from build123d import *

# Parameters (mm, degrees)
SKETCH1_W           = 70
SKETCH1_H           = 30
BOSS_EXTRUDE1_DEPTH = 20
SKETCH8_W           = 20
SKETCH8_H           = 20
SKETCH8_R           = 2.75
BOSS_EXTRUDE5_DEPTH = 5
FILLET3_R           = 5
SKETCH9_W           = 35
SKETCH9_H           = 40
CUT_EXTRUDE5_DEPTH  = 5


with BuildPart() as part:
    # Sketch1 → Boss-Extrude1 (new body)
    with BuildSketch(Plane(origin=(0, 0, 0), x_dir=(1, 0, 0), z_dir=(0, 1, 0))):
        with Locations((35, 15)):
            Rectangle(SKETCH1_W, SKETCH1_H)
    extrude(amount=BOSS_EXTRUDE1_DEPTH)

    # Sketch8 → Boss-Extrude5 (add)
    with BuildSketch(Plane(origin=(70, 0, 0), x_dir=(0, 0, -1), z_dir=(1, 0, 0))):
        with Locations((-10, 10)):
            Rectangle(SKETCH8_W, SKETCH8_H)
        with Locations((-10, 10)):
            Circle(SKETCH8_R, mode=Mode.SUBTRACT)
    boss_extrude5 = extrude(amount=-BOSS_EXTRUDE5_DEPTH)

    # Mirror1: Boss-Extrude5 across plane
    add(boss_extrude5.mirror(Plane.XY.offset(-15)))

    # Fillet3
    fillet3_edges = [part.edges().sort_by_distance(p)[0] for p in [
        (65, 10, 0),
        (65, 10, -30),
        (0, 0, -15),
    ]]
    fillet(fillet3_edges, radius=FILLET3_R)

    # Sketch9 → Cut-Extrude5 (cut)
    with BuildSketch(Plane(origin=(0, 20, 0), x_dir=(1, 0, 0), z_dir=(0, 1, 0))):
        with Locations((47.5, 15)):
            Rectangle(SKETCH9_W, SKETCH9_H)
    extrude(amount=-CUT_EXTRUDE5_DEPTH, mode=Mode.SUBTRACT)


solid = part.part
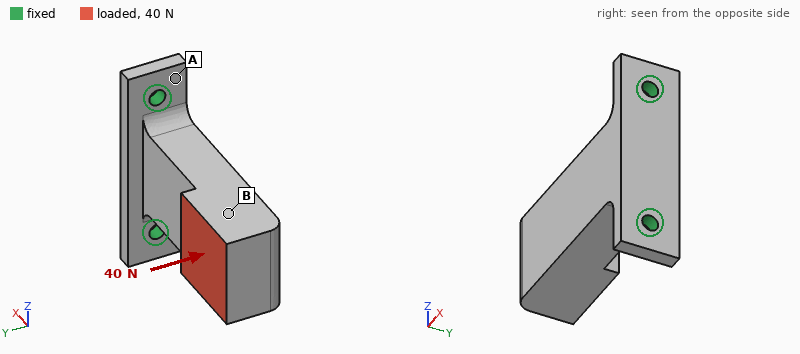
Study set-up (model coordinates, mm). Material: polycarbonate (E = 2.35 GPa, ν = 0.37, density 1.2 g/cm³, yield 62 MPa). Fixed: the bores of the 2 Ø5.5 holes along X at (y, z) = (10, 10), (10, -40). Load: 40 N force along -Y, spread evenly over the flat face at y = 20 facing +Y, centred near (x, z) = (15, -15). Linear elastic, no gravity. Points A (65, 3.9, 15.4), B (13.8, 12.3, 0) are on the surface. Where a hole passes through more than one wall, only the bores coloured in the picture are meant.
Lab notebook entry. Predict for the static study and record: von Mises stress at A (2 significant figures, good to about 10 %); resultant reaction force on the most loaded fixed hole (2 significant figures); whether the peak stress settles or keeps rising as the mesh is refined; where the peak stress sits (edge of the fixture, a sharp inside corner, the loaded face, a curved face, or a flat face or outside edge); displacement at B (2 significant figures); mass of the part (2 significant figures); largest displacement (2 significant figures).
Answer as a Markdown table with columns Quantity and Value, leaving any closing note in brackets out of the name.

| Quantity | Value |
|---|---|
| von Mises stress at A | 2.3 MPa |
| resultant reaction force on the most loaded fixed hole | 20 N |
| whether the peak stress settles or keeps rising as the mesh is refined | keeps rising |
| where the peak stress sits | edge of the fixture |
| displacement at B | 0.74 mm |
| mass of the part | 49 g |
| largest displacement | 0.95 mm |
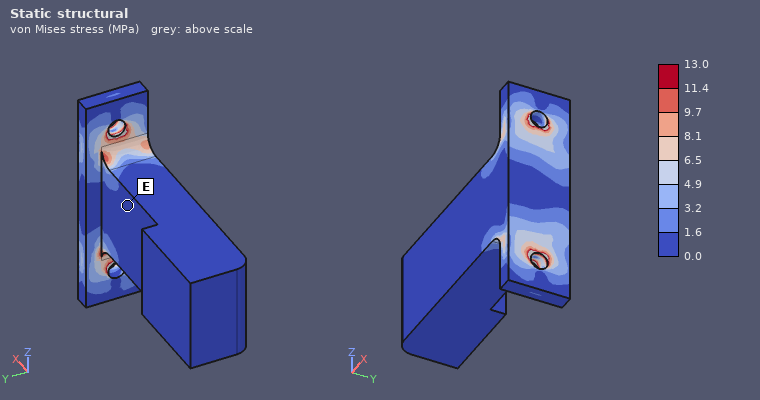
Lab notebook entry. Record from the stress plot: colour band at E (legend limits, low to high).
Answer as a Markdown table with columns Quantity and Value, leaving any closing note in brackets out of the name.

| Quantity | Value |
|---|---|
| colour band at E | 0.0 to 1.6 MPa |
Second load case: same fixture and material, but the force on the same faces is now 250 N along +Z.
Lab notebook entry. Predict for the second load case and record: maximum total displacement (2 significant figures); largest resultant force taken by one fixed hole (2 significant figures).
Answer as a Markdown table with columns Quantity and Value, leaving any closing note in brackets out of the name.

| Quantity | Value |
|---|---|
| maximum total displacement | 0.70 mm |
| largest resultant force taken by one fixed hole | 350 N |
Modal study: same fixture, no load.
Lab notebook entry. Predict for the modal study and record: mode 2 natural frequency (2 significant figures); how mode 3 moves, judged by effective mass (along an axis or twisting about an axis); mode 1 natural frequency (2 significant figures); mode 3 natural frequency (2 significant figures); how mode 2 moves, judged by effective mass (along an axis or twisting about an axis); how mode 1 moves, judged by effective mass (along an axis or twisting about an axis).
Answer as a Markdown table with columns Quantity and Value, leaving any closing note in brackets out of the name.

| Quantity | Value |
|---|---|
| mode 2 natural frequency | 750 Hz |
| how mode 3 moves, judged by effective mass | along X |
| mode 1 natural frequency | 230 Hz |
| mode 3 natural frequency | 1700 Hz |
| how mode 2 moves, judged by effective mass | along Z |
| how mode 1 moves, judged by effective mass | along Y |
